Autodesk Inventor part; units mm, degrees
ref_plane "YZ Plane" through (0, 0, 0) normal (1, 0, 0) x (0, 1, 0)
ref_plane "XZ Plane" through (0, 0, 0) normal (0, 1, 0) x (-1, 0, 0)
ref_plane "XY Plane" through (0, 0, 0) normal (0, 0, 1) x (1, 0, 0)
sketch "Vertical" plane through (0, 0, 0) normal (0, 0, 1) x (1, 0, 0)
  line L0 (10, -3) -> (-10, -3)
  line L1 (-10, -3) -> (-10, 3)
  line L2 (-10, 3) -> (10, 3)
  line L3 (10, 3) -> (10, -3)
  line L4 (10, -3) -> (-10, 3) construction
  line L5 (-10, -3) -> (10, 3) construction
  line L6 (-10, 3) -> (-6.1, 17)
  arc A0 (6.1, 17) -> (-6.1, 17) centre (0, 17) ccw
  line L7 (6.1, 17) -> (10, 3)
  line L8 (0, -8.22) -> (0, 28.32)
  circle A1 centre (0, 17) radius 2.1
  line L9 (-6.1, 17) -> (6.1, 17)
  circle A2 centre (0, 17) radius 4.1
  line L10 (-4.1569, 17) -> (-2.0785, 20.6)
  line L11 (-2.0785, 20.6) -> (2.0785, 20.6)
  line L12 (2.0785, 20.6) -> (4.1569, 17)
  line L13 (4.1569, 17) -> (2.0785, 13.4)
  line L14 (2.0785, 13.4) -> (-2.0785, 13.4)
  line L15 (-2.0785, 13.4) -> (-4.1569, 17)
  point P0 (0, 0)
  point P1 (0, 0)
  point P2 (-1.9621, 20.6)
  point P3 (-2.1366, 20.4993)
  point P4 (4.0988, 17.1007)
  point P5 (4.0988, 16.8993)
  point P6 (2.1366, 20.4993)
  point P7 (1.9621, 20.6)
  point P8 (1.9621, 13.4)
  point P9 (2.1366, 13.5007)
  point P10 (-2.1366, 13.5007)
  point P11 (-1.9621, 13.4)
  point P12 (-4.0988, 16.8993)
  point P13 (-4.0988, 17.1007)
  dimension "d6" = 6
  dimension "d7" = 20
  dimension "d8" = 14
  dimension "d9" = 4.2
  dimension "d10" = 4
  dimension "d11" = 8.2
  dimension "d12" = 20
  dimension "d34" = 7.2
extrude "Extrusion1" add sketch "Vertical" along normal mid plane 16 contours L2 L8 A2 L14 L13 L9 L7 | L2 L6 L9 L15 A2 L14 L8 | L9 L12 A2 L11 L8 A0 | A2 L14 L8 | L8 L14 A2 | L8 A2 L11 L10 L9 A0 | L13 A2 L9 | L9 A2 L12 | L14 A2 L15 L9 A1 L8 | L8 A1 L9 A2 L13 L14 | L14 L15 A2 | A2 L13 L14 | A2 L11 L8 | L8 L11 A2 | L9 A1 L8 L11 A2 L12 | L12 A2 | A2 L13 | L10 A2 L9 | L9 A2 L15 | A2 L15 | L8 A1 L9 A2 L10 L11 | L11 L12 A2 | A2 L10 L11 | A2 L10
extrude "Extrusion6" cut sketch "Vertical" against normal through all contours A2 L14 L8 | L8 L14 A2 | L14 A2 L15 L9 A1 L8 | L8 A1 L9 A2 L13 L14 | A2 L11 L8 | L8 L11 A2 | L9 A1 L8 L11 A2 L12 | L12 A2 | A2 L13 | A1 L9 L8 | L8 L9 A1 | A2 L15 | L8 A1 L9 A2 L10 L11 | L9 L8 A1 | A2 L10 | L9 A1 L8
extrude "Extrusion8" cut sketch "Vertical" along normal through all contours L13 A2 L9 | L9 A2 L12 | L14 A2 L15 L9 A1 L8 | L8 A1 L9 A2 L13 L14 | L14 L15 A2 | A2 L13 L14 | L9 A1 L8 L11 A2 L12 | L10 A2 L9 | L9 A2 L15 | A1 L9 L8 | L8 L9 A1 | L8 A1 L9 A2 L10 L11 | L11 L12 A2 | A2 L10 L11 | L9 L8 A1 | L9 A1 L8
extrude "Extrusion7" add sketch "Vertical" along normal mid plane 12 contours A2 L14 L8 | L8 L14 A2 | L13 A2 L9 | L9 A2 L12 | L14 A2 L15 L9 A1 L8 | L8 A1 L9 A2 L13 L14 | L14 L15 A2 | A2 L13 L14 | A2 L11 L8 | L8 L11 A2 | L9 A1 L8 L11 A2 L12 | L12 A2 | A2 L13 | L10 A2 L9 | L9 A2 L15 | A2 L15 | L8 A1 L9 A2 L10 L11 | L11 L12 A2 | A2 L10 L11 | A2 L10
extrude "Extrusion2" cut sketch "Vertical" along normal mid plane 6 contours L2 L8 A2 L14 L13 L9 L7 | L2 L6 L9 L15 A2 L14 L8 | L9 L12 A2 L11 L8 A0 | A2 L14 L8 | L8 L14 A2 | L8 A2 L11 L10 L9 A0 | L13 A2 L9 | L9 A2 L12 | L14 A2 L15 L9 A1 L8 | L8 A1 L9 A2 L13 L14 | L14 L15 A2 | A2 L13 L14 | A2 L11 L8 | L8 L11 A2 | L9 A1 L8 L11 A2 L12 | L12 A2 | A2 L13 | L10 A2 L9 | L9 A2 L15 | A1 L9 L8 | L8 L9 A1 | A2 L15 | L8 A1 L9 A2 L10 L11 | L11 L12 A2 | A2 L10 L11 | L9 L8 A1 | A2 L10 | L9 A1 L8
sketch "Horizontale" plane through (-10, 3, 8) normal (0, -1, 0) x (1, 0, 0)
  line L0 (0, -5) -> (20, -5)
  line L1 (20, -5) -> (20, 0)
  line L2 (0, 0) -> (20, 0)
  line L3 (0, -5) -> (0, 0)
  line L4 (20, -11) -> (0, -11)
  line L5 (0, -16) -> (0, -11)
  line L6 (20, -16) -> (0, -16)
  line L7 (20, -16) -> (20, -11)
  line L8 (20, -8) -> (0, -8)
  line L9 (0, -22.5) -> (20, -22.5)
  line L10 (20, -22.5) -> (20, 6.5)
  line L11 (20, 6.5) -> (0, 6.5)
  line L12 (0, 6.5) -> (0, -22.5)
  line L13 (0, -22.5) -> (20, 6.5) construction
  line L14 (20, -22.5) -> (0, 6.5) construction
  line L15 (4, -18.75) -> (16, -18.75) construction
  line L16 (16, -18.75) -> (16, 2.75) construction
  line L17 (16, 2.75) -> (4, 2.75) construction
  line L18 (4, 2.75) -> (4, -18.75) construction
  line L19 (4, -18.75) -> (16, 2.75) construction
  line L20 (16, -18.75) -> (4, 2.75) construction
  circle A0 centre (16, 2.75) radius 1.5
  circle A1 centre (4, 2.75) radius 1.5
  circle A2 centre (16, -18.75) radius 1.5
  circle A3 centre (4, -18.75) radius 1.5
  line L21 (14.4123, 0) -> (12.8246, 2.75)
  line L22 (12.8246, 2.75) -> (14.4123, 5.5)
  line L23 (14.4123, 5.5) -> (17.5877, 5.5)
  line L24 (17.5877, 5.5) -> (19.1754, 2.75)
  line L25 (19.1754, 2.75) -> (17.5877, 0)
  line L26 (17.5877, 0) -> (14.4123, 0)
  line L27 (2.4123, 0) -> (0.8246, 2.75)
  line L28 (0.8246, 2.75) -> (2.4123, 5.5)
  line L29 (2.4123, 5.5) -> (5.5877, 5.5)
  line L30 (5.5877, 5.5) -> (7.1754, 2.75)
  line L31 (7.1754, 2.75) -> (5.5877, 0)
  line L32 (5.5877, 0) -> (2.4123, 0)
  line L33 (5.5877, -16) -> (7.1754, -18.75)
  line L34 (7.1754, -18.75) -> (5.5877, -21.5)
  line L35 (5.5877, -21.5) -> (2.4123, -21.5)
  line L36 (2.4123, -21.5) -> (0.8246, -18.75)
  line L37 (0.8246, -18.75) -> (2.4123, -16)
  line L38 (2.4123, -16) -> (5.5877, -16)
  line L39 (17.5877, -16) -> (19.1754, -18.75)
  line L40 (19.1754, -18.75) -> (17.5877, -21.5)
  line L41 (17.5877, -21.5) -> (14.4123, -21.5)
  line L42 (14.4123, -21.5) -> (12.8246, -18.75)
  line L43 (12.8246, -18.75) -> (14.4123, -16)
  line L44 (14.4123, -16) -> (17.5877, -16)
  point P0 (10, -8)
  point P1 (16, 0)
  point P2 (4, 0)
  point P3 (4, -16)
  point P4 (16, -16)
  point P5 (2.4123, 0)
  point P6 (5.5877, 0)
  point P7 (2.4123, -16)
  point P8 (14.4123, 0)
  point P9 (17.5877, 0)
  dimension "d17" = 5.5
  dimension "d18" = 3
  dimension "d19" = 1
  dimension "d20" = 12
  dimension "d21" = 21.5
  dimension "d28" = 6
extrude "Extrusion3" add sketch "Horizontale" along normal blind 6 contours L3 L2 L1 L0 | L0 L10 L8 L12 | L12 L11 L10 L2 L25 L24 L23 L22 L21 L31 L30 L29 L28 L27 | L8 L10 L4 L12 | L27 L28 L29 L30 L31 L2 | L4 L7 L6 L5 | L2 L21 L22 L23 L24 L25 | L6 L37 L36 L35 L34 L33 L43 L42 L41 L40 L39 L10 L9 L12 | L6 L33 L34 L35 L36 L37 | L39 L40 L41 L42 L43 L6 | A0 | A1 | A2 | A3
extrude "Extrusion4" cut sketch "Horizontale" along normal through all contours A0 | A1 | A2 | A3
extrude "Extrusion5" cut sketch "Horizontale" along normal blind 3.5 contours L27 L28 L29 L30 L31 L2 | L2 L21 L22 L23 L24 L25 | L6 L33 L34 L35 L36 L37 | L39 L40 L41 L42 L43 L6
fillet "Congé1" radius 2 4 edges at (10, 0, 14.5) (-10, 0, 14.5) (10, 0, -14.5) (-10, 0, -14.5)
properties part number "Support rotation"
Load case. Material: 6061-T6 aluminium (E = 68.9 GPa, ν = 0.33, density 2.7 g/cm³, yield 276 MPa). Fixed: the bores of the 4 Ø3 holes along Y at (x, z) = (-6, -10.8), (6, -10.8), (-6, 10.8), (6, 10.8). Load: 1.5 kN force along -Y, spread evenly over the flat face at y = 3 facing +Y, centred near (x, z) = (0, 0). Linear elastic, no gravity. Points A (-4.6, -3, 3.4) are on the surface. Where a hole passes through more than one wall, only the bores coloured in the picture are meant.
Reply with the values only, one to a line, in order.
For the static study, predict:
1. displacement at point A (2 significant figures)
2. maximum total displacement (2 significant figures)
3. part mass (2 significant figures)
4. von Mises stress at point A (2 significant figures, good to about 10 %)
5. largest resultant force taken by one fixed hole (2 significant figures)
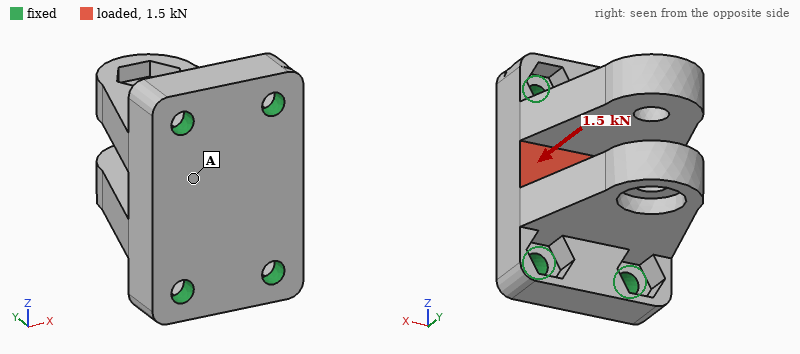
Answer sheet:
6.4 µm
18 µm
15 g
16 MPa
490 N
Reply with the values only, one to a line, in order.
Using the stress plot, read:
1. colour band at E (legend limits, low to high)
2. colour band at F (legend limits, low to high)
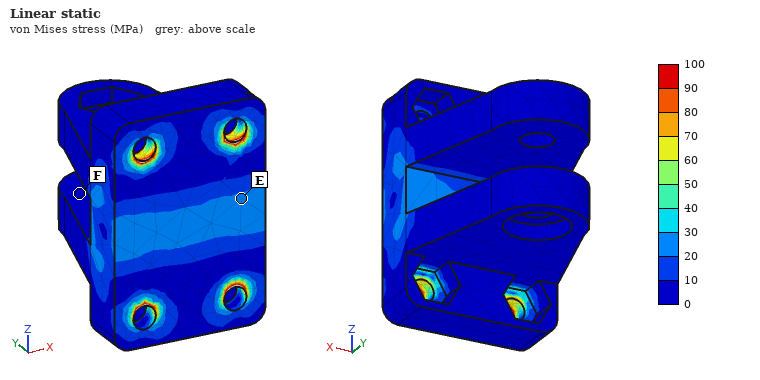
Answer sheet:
20 to 30 MPa
0 to 10 MPa
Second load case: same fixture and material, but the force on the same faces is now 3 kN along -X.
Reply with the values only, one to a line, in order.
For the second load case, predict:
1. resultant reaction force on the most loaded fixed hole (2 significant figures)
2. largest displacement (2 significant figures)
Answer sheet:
1.0 kN
20 µm
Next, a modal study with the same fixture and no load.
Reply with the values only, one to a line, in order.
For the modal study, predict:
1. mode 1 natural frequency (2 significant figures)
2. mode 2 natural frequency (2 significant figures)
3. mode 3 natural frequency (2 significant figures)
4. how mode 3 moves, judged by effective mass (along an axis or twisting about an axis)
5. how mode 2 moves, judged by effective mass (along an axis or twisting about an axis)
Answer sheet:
10 kHz
12 kHz
15 kHz
along X
along Z
